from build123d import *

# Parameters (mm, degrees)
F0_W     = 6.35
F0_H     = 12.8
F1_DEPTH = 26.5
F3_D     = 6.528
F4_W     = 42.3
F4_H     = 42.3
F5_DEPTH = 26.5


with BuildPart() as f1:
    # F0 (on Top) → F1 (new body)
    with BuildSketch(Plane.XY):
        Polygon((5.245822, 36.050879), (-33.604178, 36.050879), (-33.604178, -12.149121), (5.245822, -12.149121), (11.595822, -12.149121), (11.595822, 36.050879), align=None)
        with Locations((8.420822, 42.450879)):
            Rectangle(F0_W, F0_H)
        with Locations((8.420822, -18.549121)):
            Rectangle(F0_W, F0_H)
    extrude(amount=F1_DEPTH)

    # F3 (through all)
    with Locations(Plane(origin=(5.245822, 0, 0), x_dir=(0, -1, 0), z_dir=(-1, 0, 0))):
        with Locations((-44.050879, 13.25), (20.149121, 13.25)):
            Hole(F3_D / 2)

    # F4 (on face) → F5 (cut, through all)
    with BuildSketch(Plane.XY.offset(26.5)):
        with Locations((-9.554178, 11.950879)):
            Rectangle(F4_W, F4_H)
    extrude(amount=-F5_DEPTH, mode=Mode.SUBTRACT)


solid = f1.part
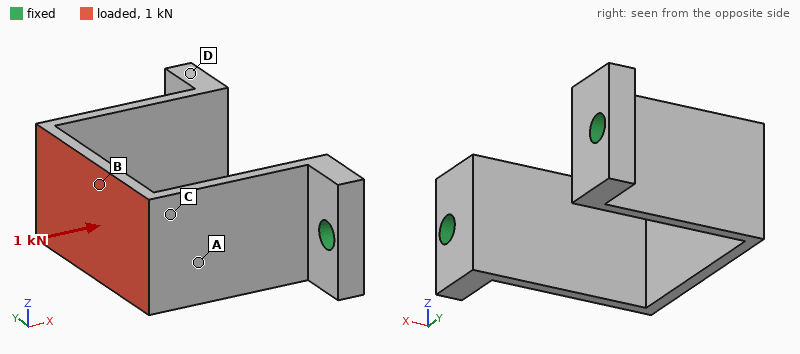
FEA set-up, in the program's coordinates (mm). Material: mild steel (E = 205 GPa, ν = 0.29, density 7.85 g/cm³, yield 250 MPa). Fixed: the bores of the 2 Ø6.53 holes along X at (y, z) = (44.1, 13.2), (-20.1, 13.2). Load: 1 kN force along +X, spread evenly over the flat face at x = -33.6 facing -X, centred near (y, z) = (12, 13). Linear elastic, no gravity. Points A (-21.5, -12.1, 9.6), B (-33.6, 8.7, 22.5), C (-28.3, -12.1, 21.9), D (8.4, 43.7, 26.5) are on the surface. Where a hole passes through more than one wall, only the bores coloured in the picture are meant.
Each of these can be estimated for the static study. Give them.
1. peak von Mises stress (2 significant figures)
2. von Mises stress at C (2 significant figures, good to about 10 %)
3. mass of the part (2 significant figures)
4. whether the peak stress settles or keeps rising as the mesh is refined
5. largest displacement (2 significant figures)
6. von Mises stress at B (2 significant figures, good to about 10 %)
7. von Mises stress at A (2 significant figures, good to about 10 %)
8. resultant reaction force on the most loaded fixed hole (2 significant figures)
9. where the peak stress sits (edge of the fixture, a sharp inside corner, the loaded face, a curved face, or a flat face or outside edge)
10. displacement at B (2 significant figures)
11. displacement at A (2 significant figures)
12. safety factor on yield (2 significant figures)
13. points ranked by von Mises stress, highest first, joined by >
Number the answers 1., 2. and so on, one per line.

1. 74 MPa
2. 48 MPa
3. 110 g
4. settles
5. 45 µm
6. 68 MPa
7. 29 MPa
8. 510 N
9. the loaded face
10. 42 µm
11. 11 µm
12. 3.4
13. B > C > A > D
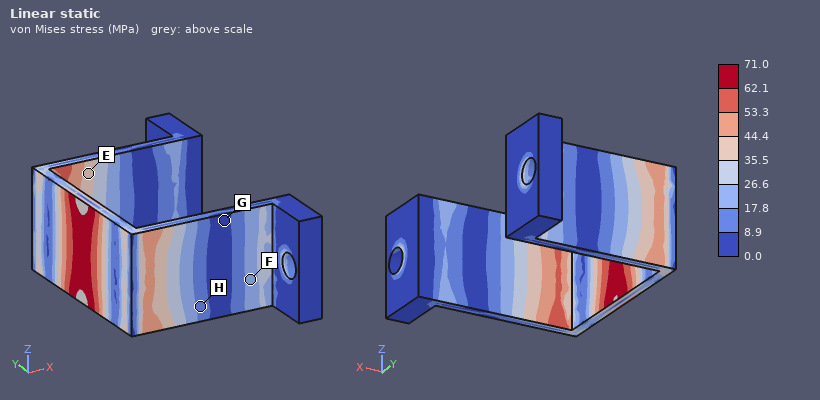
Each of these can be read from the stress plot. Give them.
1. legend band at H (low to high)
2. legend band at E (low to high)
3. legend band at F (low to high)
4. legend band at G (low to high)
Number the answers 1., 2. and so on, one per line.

1. 8.9 to 17.8 MPa
2. 35.5 to 44.4 MPa
3. 17.8 to 26.6 MPa
4. 0.0 to 8.9 MPa
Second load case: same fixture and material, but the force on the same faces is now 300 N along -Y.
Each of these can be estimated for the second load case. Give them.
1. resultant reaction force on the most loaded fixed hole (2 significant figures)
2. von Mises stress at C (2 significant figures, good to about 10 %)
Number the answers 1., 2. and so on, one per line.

1. 190 N
2. 45 MPa
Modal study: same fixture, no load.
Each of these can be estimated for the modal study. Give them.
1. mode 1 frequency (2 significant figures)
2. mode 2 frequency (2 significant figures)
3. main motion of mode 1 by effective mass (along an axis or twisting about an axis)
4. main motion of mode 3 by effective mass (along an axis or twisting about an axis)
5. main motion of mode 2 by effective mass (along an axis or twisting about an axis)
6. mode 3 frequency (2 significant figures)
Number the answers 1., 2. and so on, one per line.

1. 1400 Hz
2. 3000 Hz
3. along Y
4. twisting about X
5. along Z
6. 3800 Hz
